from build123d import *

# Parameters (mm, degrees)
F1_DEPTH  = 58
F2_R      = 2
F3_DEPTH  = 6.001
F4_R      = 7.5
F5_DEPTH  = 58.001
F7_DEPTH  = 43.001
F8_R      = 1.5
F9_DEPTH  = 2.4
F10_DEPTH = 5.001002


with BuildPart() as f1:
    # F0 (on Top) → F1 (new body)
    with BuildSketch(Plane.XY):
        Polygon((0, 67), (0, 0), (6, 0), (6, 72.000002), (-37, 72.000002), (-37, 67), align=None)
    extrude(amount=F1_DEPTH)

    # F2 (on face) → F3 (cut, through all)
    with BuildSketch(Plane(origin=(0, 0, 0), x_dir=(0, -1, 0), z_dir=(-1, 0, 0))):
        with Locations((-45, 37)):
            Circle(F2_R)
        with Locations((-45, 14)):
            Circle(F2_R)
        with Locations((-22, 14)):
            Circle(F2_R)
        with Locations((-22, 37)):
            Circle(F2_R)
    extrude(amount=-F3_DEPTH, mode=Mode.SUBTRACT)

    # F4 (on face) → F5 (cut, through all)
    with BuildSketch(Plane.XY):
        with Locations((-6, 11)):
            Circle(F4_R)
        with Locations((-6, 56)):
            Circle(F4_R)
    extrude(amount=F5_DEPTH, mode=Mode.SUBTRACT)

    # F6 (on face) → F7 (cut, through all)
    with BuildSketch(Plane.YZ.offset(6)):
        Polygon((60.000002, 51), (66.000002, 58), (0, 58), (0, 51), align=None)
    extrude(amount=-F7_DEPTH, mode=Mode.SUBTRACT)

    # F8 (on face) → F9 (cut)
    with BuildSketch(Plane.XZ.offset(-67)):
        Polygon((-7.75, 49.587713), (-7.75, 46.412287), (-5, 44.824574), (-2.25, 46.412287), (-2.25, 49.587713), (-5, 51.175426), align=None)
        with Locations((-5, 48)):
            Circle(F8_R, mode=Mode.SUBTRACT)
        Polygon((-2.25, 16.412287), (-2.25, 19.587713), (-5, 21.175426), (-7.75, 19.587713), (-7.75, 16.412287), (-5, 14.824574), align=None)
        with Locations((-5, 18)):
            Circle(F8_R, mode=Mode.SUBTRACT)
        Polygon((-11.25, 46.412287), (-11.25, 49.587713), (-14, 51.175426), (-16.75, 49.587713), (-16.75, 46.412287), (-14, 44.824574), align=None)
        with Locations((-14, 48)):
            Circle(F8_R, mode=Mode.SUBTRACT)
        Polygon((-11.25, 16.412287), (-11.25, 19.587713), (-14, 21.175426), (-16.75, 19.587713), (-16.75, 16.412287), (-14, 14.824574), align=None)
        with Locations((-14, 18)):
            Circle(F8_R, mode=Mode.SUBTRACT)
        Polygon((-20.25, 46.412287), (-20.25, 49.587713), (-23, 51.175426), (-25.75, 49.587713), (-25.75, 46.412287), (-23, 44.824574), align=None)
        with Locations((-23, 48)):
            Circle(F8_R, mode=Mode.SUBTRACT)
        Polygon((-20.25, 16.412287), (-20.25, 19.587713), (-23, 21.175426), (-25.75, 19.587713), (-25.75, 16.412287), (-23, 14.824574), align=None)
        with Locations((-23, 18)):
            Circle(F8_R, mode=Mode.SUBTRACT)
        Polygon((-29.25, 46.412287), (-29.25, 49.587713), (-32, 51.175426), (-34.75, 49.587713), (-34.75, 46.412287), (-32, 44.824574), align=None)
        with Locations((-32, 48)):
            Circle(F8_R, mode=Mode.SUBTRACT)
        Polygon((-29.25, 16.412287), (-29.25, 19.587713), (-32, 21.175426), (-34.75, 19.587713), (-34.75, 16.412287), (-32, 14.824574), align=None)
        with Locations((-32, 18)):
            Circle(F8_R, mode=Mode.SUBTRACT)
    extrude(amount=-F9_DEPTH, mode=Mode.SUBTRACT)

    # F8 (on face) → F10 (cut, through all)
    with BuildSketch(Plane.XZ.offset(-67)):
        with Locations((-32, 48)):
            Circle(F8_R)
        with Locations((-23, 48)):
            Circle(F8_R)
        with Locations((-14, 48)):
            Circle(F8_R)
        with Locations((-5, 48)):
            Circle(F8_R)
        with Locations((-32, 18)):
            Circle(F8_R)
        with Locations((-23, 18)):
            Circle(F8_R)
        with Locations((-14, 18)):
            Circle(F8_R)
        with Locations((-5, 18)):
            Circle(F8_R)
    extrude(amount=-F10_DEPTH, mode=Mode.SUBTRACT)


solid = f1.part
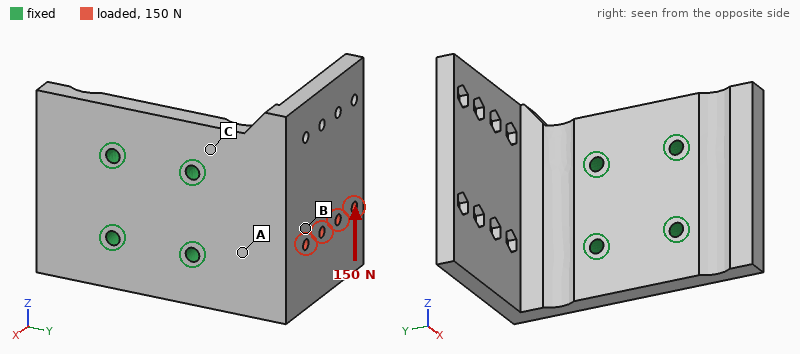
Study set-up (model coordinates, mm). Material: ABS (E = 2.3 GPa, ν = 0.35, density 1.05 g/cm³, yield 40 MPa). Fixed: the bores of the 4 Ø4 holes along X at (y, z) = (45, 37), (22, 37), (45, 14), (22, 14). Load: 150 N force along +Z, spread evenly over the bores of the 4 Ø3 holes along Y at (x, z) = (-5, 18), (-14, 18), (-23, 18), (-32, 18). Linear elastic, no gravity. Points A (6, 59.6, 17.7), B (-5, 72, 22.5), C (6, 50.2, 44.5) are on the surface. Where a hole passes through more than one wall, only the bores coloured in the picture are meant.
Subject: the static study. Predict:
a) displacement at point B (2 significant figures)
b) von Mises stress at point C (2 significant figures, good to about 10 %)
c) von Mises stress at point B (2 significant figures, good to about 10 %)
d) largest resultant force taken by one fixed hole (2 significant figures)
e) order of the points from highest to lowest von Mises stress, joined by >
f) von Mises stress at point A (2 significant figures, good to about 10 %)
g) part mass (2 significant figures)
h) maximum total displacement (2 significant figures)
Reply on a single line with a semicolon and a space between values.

0.16 mm; 6.4 MPa; 1.2 MPa; 170 N; C > A > B; 4.3 MPa; 33 g; 0.86 mm
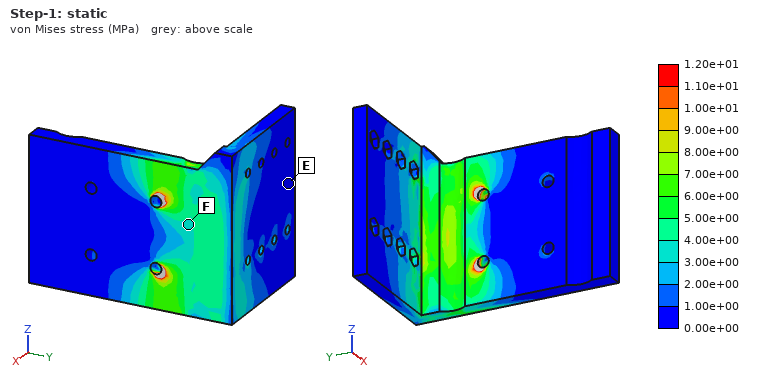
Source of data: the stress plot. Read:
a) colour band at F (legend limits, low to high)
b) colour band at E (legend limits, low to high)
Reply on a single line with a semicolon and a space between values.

3.00e+00 to 4.00e+00 MPa; 0.00e+00 to 1.00e+00 MPa
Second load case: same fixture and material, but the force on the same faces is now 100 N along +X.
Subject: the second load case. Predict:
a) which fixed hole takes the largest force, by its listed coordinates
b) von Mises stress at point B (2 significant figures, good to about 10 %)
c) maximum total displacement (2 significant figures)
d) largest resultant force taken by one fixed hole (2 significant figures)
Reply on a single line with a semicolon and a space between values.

(45, 14); 1.2 MPa; 1.1 mm; 97 N
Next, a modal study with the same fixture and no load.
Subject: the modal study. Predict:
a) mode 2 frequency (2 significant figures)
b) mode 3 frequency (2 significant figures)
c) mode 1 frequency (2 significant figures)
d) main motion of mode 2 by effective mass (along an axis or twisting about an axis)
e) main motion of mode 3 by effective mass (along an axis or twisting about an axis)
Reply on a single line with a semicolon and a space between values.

690 Hz; 1200 Hz; 400 Hz; along Z; along X
